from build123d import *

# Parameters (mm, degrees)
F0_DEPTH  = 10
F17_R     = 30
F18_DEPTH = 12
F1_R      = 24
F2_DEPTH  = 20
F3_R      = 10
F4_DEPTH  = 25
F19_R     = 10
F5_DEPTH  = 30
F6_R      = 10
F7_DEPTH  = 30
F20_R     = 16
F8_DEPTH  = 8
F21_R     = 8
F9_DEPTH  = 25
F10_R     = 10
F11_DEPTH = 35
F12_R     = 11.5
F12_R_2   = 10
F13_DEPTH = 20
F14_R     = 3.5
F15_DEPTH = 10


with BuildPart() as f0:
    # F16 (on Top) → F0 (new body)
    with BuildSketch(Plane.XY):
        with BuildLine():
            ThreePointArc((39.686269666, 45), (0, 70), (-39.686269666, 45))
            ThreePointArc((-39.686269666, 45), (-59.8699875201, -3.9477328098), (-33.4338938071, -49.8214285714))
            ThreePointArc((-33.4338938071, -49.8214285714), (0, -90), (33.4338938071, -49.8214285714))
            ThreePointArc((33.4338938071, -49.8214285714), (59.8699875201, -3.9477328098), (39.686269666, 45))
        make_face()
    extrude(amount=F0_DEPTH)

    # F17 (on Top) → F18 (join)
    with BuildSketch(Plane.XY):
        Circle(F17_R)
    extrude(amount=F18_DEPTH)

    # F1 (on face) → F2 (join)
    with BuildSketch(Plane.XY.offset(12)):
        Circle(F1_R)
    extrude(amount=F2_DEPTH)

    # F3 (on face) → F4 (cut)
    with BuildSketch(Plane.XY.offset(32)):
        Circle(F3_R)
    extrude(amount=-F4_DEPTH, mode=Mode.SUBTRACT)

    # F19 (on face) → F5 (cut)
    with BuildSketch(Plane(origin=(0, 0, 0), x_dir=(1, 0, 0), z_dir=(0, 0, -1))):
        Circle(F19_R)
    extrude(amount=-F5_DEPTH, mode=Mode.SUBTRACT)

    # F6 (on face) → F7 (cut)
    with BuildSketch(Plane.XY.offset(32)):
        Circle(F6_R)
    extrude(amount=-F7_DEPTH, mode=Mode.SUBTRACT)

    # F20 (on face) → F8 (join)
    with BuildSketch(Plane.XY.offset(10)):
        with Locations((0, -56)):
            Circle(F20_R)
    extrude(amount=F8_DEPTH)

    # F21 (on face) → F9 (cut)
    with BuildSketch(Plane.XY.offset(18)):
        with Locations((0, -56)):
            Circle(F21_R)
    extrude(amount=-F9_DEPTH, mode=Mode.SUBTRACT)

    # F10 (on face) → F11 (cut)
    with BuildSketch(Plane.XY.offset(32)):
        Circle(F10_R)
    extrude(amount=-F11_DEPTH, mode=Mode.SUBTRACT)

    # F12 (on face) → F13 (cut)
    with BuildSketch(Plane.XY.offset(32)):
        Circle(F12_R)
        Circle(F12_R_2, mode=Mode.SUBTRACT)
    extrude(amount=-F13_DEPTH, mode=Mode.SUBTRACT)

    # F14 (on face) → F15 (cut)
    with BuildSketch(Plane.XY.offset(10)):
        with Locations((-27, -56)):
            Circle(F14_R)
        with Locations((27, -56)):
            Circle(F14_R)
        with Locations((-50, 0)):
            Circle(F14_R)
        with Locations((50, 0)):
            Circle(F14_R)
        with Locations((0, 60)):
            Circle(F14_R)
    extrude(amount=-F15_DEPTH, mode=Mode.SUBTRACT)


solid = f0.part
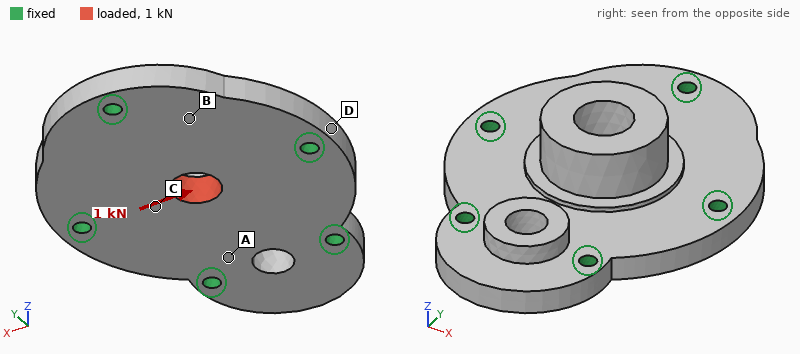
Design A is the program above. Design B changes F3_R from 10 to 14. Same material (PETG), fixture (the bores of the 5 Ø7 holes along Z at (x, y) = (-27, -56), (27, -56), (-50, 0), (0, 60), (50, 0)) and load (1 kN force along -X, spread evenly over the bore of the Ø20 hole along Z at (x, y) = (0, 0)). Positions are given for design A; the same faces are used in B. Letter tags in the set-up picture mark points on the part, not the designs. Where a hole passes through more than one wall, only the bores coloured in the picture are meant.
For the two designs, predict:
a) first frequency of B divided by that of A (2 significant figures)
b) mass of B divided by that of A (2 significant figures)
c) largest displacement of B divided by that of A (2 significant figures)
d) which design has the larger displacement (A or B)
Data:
1.0
0.97
1.2
B
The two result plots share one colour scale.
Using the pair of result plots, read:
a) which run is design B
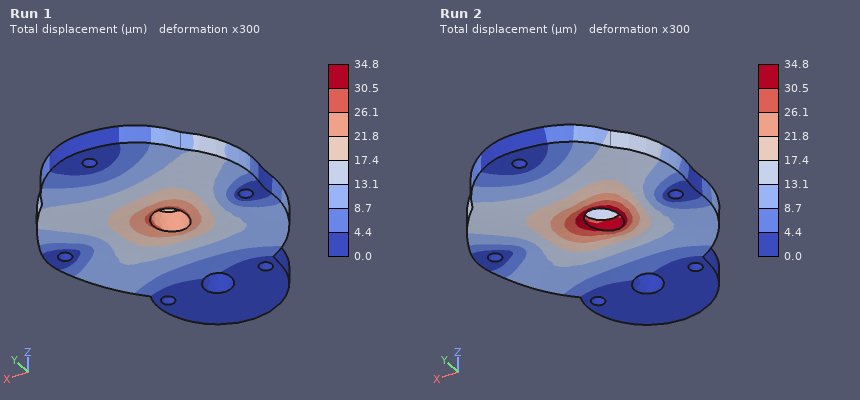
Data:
Run 2
